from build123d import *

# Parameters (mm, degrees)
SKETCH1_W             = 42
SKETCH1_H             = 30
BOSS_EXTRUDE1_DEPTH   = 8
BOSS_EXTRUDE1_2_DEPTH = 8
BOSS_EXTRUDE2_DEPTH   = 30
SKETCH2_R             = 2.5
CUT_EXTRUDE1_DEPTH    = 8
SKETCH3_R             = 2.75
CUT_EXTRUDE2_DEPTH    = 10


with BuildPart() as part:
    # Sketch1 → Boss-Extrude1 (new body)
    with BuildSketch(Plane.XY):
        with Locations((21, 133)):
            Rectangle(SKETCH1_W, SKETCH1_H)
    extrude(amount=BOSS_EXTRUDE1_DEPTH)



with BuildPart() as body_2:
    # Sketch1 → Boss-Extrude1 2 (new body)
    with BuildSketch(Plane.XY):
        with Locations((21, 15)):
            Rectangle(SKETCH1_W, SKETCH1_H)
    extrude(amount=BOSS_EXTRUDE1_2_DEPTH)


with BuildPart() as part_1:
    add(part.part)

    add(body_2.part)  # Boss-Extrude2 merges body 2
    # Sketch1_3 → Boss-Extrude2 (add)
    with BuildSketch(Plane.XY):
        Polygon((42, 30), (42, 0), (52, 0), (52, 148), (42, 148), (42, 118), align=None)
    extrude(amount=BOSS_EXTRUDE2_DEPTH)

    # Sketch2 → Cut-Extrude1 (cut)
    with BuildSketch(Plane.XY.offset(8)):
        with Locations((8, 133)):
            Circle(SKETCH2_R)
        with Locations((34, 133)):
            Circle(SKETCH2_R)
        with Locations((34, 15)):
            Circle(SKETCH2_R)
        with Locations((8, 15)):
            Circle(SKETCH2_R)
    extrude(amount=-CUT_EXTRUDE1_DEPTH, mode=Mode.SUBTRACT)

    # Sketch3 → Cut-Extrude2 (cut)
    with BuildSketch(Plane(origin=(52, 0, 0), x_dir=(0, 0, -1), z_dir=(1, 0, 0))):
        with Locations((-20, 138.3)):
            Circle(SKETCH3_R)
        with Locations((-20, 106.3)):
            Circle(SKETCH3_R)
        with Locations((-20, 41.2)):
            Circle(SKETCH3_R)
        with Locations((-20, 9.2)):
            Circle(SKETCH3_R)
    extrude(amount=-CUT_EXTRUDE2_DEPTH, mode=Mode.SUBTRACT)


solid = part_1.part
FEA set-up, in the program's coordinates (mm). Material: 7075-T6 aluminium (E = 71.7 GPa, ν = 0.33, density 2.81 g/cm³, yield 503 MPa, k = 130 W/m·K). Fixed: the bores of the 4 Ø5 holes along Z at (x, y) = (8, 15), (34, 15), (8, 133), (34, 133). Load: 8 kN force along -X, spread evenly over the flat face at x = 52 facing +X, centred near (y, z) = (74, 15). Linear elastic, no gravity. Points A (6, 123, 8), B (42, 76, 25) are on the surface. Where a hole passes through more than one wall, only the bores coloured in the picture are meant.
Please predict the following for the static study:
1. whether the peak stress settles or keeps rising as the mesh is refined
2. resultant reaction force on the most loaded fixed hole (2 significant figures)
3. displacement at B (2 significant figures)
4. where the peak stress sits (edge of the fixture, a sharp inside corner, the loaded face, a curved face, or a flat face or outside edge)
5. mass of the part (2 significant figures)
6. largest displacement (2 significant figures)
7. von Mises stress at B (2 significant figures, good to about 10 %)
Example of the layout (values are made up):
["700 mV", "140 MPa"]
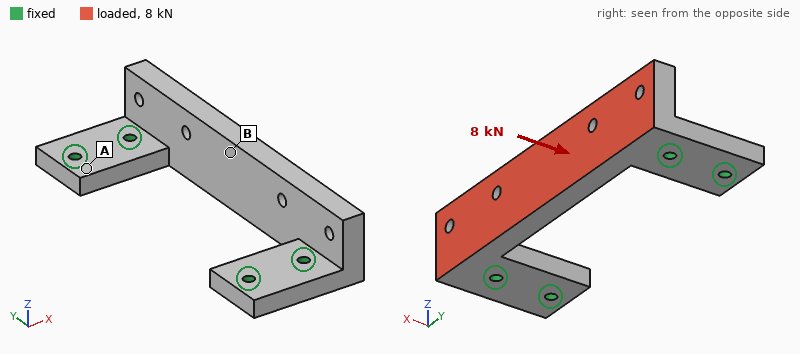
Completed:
["keeps rising", "3.2 kN", "0.30 mm", "edge of the fixture", "180 g", "0.36 mm", "61 MPa"]
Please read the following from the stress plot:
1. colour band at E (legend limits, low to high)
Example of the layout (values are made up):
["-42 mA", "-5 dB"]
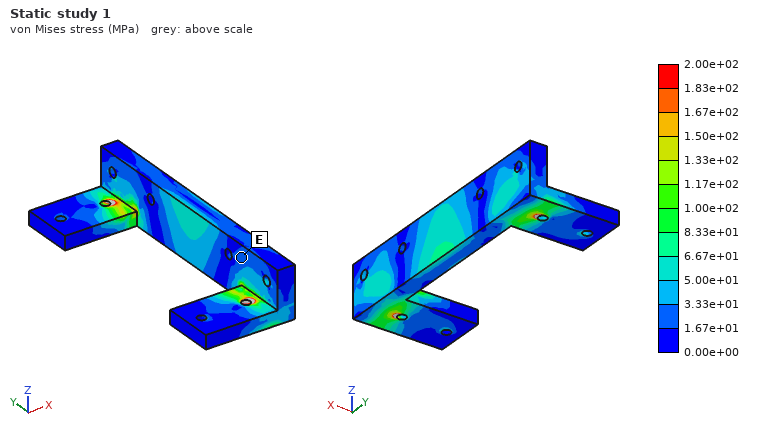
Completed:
["1.67e+01 to 3.33e+01 MPa"]
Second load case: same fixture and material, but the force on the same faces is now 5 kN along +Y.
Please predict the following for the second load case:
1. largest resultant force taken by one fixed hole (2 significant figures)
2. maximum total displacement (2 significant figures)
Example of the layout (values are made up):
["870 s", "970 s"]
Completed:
["3.3 kN", "23 µm"]
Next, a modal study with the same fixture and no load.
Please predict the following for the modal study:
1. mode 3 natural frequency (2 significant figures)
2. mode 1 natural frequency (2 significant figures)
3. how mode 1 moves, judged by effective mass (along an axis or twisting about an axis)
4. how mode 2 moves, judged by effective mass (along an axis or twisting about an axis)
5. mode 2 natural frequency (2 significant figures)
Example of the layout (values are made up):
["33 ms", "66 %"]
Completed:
["5300 Hz", "2700 Hz", "along X", "along Z", "4800 Hz"]
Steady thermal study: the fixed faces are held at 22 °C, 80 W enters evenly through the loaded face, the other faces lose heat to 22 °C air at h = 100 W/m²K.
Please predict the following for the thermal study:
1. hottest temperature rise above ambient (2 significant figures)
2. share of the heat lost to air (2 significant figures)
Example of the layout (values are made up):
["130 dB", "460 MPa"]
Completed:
["31 K", "25 %"]
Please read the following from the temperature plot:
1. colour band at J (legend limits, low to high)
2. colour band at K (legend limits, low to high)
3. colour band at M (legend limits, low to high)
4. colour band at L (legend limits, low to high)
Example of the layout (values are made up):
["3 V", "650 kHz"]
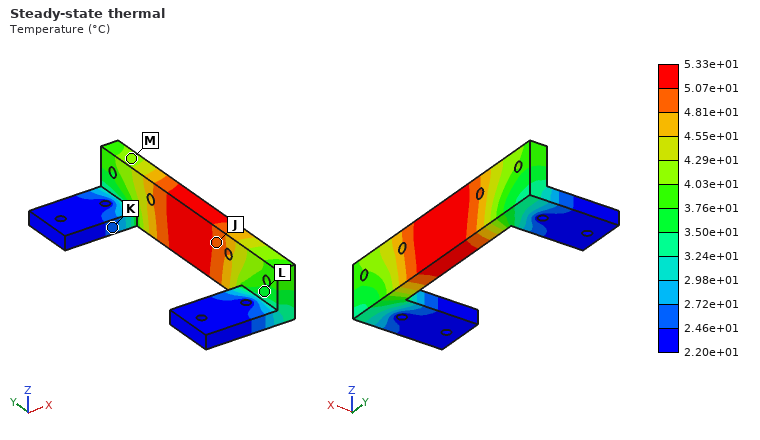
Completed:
["4.81e+01 to 5.07e+01 °C", "2.46e+01 to 2.72e+01 °C", "4.03e+01 to 4.29e+01 °C", "3.50e+01 to 3.76e+01 °C"]
